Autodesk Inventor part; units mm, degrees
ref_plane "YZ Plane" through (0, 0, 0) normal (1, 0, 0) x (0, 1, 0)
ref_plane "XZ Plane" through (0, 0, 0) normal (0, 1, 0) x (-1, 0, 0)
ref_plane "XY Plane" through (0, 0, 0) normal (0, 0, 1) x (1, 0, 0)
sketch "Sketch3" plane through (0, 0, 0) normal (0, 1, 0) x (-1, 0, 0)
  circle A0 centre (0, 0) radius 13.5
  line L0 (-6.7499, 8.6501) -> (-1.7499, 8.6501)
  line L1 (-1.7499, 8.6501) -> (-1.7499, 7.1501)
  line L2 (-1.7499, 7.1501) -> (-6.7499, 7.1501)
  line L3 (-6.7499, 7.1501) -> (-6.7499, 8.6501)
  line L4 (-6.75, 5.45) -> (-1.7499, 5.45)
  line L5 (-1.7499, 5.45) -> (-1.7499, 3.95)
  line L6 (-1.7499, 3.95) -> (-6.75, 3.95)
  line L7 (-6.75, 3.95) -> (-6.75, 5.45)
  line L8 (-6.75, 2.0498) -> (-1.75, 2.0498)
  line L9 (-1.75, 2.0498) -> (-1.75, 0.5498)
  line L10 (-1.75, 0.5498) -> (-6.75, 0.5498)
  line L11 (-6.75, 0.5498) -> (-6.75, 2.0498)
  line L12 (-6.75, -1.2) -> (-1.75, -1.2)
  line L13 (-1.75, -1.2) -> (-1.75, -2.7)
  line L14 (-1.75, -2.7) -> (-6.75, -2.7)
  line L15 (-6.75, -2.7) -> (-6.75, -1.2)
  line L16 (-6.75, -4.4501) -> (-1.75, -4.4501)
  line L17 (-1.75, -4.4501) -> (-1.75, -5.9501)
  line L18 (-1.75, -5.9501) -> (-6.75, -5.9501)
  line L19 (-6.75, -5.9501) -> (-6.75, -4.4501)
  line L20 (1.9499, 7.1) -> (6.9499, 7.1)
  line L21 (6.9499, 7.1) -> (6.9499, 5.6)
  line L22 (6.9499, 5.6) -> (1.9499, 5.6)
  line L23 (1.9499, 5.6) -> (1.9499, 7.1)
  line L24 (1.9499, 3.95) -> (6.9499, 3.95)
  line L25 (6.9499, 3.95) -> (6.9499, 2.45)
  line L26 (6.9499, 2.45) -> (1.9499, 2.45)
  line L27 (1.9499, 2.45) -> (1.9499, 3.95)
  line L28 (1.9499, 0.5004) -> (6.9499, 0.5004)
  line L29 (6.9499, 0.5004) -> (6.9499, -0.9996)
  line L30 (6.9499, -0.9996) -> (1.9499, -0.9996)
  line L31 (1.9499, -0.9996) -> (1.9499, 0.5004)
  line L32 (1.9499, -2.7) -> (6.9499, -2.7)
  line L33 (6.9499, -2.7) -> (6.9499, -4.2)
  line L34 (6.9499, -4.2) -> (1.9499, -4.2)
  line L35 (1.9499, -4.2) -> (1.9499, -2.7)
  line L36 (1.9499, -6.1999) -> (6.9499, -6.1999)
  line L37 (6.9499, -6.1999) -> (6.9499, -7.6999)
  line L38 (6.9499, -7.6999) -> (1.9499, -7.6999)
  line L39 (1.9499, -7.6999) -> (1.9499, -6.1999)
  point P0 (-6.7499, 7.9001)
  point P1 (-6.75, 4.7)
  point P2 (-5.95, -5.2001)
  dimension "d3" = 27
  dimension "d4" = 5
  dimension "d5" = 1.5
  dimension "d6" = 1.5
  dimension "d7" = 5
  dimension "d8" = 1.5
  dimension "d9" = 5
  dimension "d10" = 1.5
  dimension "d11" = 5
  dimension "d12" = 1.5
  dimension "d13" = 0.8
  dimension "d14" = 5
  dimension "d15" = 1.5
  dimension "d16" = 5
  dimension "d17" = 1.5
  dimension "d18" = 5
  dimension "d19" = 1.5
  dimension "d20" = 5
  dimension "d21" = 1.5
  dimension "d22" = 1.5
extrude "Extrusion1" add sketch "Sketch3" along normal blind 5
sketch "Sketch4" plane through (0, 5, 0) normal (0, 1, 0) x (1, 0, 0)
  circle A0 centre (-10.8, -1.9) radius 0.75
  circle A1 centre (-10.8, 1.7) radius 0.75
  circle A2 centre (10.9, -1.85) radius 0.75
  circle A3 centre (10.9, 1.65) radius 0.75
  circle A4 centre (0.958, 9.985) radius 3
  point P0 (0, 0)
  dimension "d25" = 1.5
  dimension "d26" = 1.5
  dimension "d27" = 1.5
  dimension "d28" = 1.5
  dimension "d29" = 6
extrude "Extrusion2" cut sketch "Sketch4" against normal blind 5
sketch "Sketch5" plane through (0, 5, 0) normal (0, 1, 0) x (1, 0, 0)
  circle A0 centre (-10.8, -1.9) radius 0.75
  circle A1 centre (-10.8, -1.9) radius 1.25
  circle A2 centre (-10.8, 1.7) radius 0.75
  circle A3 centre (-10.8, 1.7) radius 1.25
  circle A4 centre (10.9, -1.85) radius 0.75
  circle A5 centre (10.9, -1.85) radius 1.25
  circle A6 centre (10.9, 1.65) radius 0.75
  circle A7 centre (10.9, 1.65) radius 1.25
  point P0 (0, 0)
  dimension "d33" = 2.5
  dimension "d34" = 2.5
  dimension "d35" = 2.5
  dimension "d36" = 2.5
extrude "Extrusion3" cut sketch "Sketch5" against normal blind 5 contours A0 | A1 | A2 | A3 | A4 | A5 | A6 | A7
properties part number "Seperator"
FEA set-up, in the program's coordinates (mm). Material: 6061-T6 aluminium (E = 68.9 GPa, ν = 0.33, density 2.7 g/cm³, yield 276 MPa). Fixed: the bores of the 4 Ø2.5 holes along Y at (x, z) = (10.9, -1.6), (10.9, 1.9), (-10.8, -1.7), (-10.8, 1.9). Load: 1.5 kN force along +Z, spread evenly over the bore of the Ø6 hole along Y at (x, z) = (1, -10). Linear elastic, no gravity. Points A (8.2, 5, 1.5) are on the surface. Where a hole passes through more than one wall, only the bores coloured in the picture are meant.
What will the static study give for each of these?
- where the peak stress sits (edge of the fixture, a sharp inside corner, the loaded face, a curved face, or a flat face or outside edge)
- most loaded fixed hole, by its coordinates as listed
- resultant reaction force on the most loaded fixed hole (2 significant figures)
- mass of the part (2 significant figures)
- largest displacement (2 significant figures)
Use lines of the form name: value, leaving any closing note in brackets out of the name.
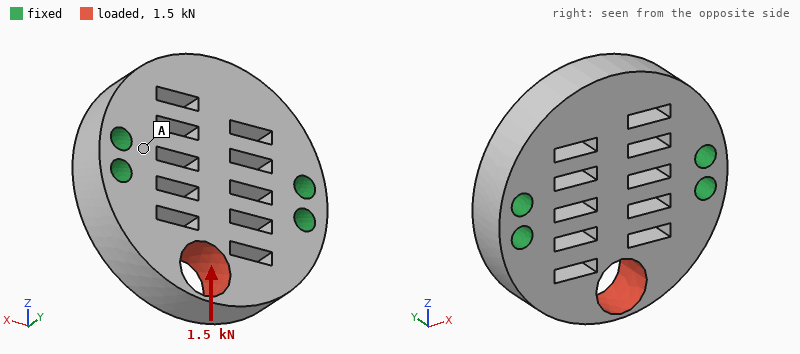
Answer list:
where the peak stress sits: a curved face
most loaded fixed hole, by its coordinates as listed: (10.9, -1.6)
resultant reaction force on the most loaded fixed hole: 580 N
mass of the part: 6.1 g
largest displacement: 18 µm
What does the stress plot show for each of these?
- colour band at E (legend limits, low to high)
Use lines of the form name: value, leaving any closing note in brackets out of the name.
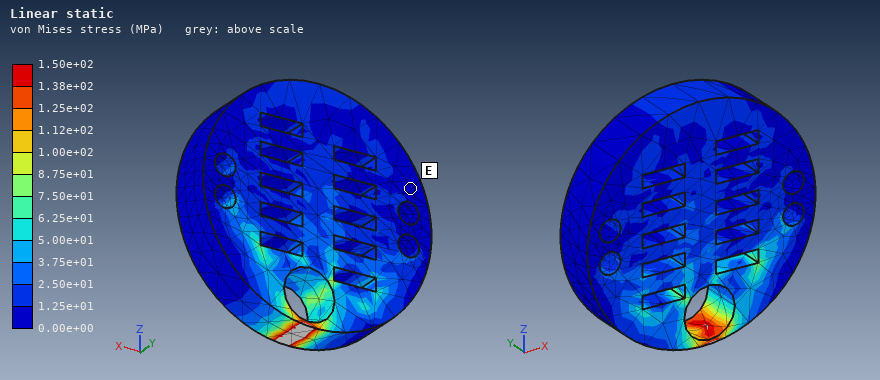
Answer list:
colour band at E: 0.00e+00 to 1.25e+01 MPa
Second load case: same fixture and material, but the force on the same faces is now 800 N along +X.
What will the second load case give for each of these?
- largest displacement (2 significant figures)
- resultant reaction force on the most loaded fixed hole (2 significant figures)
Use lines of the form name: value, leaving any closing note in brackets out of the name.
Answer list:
largest displacement: 9.7 µm
resultant reaction force on the most loaded fixed hole: 500 N
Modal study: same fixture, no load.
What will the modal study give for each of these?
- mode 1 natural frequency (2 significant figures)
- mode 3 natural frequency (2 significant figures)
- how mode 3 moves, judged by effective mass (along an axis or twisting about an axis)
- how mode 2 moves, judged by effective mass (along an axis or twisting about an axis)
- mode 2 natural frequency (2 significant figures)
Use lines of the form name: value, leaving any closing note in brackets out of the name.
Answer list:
mode 1 natural frequency: 22 kHz
mode 3 natural frequency: 42 kHz
how mode 3 moves, judged by effective mass: along Z
how mode 2 moves, judged by effective mass: along Y
mode 2 natural frequency: 26 kHz
